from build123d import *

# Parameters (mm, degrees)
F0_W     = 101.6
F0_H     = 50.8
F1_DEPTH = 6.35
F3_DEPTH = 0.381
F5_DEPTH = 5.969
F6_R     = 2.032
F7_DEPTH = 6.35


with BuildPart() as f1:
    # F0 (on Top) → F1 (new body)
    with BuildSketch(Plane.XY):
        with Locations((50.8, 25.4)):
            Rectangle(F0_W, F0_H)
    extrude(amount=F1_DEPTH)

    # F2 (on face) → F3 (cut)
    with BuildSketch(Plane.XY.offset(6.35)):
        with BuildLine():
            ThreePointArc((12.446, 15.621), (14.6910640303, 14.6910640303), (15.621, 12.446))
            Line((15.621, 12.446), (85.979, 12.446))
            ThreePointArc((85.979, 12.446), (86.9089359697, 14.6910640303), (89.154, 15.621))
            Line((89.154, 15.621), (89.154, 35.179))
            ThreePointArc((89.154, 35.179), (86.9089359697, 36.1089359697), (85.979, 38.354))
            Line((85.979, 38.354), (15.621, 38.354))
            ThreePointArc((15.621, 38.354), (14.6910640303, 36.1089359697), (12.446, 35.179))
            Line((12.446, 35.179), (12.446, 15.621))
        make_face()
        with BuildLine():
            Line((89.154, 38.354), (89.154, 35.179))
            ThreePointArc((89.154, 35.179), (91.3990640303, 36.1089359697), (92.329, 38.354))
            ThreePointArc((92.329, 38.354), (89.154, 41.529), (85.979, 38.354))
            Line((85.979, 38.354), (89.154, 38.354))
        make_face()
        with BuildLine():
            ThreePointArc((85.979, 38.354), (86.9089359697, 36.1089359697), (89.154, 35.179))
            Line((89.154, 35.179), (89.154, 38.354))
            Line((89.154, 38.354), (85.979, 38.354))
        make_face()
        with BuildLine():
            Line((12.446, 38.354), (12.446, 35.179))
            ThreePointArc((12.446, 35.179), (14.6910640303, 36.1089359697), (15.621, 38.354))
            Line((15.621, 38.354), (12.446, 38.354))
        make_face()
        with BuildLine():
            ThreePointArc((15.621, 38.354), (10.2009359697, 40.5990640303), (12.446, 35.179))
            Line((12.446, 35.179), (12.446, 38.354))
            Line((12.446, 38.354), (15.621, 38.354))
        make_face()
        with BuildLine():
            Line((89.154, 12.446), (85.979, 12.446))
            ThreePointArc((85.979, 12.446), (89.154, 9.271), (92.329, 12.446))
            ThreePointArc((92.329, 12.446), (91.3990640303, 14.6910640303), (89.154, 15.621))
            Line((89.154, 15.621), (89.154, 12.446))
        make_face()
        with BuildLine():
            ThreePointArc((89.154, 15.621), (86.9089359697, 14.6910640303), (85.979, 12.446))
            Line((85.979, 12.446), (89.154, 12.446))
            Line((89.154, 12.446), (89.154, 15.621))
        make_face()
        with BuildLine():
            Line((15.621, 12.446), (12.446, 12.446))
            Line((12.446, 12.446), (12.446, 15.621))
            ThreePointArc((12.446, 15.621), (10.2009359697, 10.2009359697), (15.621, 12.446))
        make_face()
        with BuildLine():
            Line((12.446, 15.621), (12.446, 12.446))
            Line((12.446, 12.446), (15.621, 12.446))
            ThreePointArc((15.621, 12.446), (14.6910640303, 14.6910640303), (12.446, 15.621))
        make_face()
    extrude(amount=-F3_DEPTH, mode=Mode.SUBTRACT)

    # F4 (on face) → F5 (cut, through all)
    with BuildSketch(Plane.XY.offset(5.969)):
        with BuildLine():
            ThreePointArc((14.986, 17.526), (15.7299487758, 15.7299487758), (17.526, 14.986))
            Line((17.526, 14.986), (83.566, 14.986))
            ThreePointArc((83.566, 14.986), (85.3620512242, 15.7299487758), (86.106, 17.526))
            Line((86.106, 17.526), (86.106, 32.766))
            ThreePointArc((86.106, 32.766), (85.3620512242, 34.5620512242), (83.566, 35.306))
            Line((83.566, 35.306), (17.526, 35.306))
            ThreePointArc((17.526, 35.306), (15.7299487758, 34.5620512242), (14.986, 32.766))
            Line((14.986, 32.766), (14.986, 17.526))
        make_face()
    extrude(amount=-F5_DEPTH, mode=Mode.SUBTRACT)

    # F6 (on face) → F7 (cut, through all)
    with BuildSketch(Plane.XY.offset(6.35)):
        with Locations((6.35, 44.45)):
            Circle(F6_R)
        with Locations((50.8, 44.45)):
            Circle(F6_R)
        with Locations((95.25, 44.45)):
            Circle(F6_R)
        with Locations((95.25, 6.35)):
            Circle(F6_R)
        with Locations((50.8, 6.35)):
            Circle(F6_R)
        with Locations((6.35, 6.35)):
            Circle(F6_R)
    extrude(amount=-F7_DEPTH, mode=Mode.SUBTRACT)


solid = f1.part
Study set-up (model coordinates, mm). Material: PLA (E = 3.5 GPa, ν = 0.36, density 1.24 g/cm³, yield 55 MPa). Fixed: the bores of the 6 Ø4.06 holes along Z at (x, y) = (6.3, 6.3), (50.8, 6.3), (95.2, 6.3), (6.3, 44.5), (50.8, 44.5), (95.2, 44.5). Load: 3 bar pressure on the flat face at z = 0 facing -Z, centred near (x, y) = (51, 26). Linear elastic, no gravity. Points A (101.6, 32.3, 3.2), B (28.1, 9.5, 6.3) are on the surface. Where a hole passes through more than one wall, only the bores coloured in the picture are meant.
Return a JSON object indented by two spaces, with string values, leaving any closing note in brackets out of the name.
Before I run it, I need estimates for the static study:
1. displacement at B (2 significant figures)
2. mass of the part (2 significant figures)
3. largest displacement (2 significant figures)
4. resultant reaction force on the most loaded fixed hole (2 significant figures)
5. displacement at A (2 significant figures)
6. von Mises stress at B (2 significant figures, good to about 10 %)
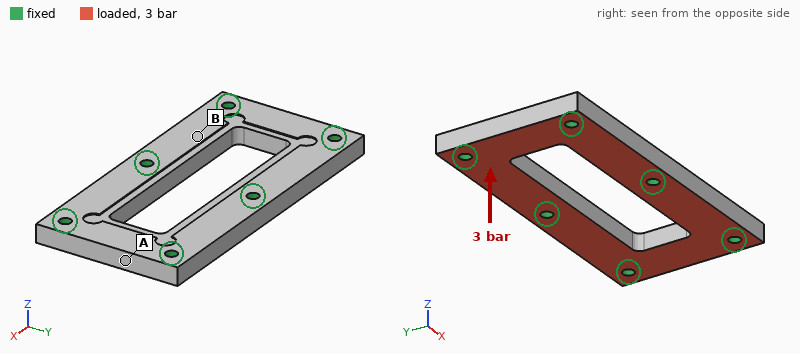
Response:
{
  "displacement at B": "50 µm",
  "mass of the part": "28 g",
  "largest displacement": "62 µm",
  "resultant reaction force on the most loaded fixed hole": "210 N",
  "displacement at A": "15 µm",
  "von Mises stress at B": "3.5 MPa"
}
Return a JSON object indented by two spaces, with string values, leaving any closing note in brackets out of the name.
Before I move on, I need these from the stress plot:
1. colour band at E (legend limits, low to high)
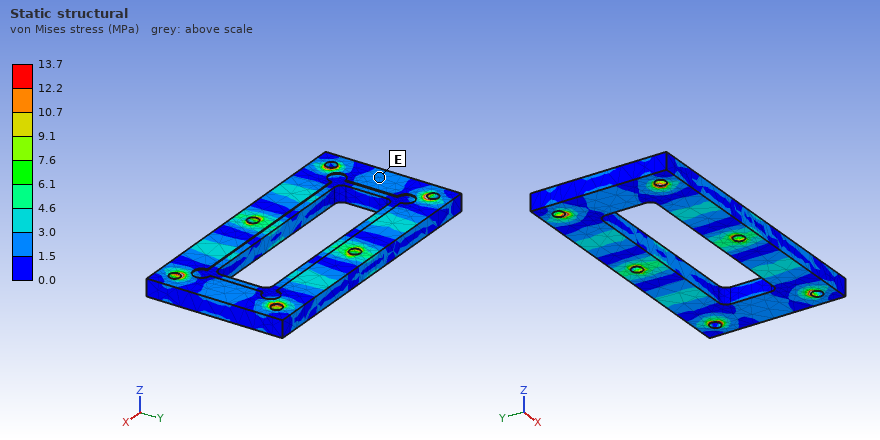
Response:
{
  "colour band at E": "1.5 to 3.0 MPa"
}
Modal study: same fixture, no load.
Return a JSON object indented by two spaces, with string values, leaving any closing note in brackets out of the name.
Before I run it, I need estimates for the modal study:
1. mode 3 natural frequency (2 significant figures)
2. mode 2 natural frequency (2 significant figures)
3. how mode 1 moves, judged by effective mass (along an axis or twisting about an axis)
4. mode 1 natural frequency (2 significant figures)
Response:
{
  "mode 3 natural frequency": "5000 Hz",
  "mode 2 natural frequency": "5000 Hz",
  "how mode 1 moves, judged by effective mass": "twisting about Y",
  "mode 1 natural frequency": "4700 Hz"
}
